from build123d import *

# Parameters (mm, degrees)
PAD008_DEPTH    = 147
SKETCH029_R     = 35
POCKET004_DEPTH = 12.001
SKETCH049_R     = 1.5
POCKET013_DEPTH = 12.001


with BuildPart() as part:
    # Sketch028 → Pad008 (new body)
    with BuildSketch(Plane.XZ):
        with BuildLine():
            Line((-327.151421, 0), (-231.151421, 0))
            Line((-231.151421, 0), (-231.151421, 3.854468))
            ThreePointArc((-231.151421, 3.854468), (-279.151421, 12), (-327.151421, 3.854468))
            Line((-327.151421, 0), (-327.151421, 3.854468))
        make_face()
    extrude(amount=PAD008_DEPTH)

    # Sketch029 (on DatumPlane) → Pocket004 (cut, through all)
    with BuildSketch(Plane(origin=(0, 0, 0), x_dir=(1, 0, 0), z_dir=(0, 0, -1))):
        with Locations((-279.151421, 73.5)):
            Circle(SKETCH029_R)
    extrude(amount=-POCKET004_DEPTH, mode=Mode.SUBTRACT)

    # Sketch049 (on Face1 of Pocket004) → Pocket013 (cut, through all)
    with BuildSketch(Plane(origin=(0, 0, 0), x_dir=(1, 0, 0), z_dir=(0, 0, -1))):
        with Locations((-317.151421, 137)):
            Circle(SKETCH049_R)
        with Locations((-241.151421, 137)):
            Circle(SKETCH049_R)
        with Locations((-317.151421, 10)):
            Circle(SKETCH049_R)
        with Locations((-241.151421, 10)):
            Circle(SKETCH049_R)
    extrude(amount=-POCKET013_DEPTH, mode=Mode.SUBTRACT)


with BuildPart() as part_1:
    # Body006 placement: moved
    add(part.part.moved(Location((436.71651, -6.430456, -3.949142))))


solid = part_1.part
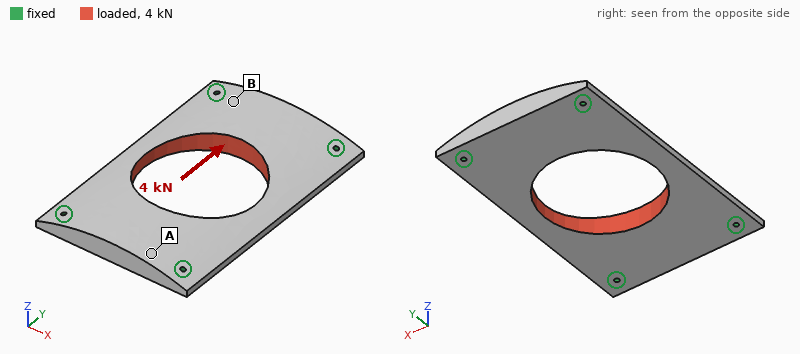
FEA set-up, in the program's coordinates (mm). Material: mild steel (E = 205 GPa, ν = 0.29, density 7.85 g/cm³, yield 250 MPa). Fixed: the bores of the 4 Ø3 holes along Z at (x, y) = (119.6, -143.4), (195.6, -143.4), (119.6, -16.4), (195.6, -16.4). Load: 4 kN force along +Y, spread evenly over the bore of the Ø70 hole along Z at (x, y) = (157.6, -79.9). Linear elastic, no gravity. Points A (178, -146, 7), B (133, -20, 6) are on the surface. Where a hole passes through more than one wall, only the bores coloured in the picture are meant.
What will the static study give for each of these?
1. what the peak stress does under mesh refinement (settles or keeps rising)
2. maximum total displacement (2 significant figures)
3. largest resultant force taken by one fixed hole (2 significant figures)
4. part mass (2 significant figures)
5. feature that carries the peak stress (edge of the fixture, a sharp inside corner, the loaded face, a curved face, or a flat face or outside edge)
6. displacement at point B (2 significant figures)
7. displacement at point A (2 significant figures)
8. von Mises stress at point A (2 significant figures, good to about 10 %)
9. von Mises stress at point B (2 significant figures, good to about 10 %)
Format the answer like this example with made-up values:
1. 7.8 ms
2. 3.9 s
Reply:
1. keeps rising
2. 1.8 µm
3. 1.0 kN
4. 700 g
5. edge of the fixture
6. 1.0 µm
7. 1.2 µm
8. 1.8 MPa
9. 3.5 MPa
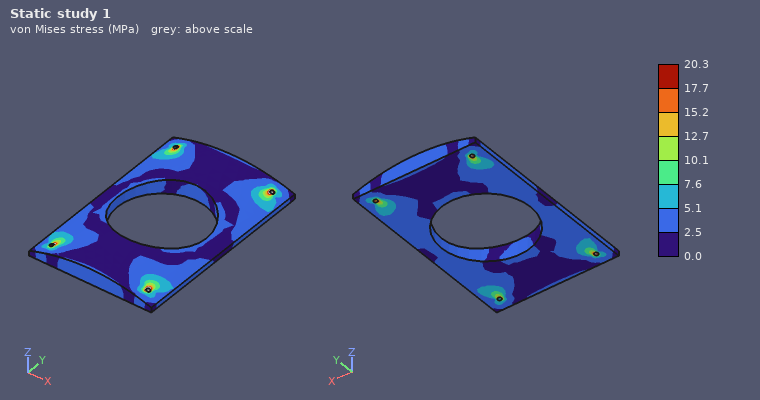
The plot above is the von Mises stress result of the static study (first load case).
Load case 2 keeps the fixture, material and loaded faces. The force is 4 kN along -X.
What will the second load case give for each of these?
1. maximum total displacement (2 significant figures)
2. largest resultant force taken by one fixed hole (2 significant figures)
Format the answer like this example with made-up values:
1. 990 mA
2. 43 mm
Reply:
1. 5.8 µm
2. 1.2 kN
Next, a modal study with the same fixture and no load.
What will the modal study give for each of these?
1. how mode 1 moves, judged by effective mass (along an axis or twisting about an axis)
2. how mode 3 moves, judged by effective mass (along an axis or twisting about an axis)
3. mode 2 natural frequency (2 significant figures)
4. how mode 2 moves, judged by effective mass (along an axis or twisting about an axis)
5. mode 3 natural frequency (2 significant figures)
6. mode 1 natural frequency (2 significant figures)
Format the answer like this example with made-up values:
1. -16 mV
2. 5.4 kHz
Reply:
1. along Z
2. twisting about X
3. 3500 Hz
4. twisting about Y
5. 4200 Hz
6. 2100 Hz
